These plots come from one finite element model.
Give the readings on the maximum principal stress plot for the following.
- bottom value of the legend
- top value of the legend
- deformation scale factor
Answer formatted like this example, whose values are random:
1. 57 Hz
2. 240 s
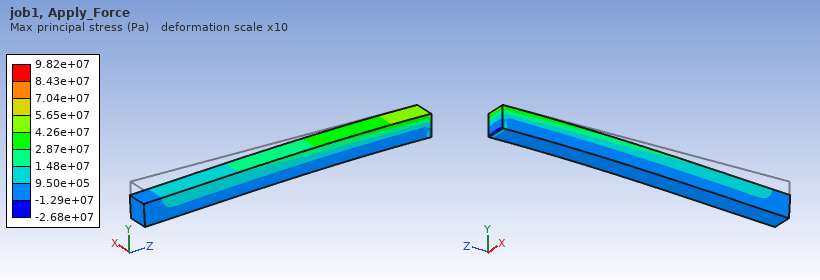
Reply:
1. -2.68e+07 Pa
2. 9.82e+07 Pa
3. 10
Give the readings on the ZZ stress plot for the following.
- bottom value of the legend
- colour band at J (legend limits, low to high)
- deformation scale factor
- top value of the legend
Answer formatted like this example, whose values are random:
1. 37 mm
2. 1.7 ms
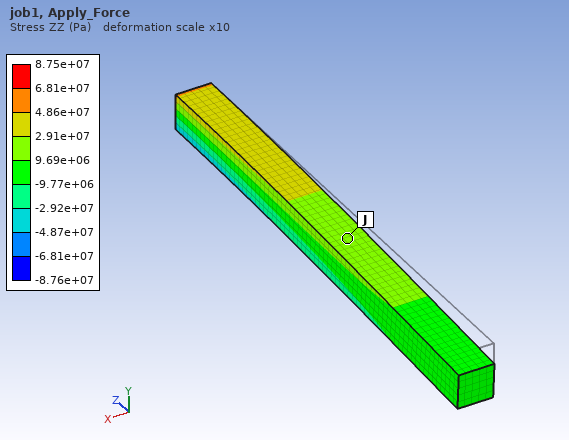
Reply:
1. -8.76e+07 Pa
2. 9.69e+06 to 2.91e+07 Pa
3. 10
4. 8.75e+07 Pa
